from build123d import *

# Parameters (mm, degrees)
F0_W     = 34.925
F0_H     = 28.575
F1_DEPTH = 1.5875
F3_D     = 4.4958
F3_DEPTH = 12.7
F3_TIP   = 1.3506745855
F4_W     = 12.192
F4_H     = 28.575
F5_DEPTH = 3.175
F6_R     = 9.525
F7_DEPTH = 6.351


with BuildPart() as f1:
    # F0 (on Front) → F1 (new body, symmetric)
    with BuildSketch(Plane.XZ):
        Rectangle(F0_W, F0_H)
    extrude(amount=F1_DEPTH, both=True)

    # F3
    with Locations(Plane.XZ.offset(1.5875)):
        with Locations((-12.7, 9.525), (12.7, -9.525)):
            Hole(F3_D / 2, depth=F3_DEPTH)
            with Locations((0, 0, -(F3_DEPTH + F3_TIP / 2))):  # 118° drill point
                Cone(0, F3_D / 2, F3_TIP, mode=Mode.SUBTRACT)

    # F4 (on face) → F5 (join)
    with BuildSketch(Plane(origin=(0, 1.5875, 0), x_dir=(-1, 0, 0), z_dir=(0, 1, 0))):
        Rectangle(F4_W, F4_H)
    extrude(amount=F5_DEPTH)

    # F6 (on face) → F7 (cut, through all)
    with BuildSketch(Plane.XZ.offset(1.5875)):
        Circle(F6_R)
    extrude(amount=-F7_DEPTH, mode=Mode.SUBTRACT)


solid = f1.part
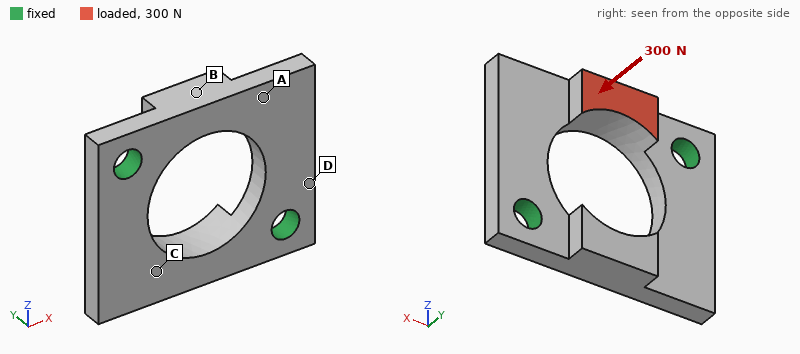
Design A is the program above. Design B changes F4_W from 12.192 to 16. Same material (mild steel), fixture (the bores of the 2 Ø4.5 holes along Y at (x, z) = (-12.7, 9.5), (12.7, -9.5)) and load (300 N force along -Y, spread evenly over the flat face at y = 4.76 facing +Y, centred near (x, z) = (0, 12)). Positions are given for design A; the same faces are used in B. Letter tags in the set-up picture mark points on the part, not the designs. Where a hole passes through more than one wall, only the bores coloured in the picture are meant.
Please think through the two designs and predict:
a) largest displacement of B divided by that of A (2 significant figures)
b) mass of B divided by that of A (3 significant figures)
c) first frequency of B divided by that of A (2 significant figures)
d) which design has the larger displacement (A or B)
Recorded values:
0.87
1.07
1.0
A
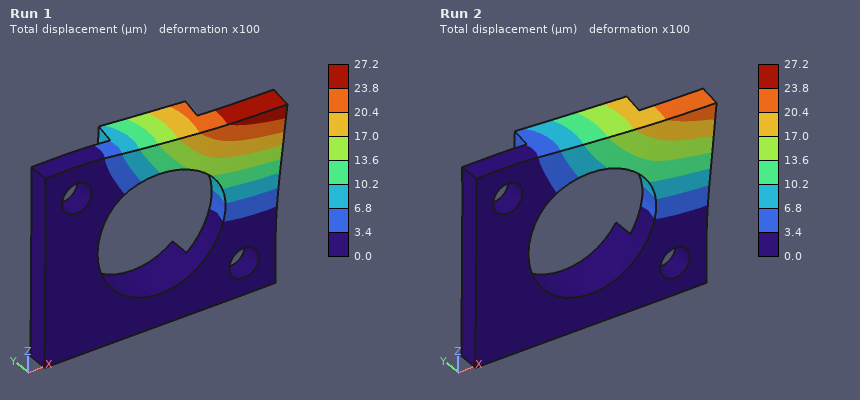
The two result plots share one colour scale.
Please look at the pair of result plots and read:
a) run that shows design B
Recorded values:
Run 2
